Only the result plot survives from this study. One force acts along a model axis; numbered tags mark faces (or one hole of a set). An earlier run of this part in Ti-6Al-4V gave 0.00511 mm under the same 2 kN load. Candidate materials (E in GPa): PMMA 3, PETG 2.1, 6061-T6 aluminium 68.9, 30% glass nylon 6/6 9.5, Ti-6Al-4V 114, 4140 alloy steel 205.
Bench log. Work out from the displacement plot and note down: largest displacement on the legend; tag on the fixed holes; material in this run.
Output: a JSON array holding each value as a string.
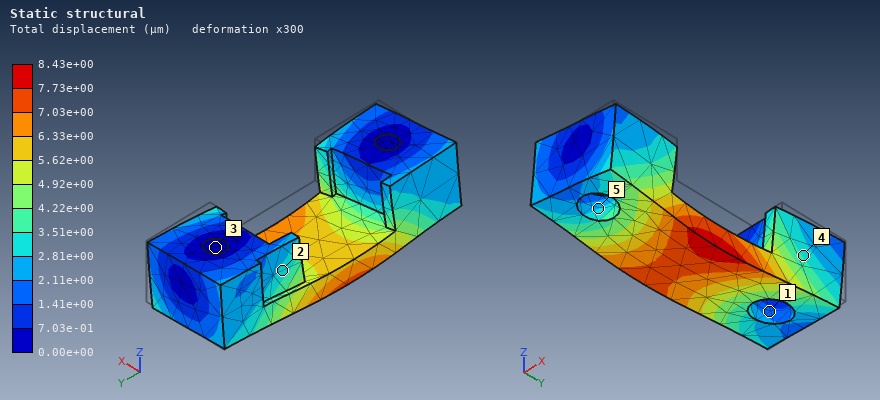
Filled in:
["8.43e+00 µm", "3", "6061-T6 aluminium"]
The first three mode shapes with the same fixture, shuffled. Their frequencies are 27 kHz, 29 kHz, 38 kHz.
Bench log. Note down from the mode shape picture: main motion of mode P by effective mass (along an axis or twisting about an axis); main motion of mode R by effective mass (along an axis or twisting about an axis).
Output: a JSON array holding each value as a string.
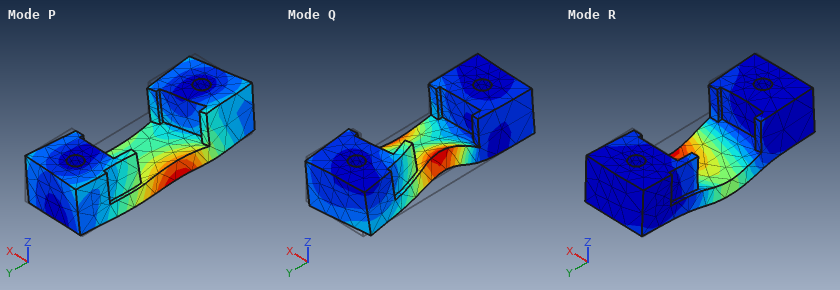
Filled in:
["along X", "along Z"]
